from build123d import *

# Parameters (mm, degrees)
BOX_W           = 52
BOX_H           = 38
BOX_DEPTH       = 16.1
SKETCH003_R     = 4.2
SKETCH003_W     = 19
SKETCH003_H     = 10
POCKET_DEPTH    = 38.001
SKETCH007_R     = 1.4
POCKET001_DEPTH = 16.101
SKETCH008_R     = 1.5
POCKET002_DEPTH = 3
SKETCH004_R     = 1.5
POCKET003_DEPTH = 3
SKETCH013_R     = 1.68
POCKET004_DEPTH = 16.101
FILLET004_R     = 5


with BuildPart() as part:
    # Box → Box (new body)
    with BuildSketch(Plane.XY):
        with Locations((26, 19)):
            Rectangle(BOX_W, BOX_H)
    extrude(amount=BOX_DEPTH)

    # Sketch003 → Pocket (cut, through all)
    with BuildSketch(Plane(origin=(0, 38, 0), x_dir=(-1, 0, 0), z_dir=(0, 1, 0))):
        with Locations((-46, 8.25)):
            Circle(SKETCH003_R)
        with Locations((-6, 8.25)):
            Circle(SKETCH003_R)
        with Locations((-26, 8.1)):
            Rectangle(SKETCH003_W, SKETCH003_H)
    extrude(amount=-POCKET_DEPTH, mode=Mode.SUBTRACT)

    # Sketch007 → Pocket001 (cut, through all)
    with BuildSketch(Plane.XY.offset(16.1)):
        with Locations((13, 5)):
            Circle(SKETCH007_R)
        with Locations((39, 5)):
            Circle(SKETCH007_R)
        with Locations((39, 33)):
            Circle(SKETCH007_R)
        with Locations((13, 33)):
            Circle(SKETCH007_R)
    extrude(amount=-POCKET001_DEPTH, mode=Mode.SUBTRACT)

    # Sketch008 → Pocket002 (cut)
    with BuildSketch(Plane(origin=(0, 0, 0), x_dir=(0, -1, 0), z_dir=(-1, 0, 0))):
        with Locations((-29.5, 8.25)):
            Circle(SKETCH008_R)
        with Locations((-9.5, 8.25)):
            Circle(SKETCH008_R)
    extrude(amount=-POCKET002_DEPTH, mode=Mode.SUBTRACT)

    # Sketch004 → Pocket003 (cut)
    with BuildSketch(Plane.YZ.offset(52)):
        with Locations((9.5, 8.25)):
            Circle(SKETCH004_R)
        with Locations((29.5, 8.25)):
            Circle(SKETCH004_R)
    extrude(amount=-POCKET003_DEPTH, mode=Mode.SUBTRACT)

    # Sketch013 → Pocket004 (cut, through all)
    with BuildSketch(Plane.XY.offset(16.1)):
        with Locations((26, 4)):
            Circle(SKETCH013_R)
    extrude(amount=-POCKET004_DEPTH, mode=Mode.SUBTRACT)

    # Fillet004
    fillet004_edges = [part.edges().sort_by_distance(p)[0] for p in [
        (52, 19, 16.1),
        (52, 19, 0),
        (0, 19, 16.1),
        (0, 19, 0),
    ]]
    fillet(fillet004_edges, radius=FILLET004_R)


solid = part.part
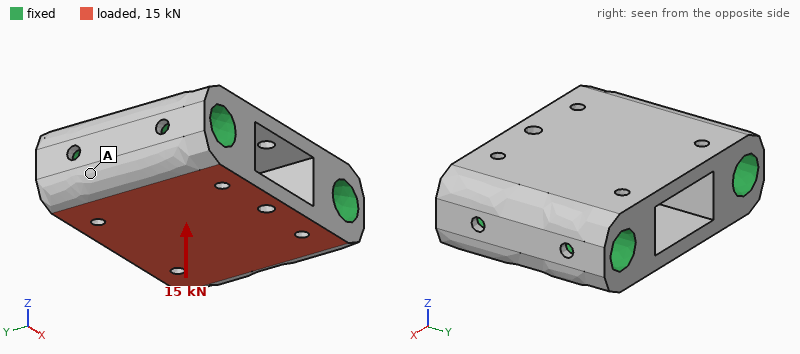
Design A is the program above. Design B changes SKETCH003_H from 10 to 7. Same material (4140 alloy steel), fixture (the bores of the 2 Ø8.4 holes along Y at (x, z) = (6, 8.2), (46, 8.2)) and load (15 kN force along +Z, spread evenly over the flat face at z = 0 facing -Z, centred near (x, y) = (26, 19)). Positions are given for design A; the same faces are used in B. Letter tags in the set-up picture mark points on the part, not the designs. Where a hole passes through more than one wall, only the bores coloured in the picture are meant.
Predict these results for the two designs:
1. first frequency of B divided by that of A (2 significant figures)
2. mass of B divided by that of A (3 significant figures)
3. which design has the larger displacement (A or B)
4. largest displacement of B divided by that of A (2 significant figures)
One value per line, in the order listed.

1.1
1.11
A
0.50
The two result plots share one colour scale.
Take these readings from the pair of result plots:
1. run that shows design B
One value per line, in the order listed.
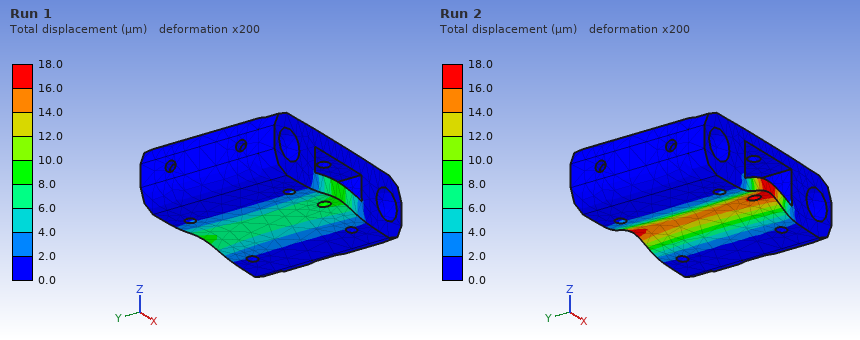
Run 1
